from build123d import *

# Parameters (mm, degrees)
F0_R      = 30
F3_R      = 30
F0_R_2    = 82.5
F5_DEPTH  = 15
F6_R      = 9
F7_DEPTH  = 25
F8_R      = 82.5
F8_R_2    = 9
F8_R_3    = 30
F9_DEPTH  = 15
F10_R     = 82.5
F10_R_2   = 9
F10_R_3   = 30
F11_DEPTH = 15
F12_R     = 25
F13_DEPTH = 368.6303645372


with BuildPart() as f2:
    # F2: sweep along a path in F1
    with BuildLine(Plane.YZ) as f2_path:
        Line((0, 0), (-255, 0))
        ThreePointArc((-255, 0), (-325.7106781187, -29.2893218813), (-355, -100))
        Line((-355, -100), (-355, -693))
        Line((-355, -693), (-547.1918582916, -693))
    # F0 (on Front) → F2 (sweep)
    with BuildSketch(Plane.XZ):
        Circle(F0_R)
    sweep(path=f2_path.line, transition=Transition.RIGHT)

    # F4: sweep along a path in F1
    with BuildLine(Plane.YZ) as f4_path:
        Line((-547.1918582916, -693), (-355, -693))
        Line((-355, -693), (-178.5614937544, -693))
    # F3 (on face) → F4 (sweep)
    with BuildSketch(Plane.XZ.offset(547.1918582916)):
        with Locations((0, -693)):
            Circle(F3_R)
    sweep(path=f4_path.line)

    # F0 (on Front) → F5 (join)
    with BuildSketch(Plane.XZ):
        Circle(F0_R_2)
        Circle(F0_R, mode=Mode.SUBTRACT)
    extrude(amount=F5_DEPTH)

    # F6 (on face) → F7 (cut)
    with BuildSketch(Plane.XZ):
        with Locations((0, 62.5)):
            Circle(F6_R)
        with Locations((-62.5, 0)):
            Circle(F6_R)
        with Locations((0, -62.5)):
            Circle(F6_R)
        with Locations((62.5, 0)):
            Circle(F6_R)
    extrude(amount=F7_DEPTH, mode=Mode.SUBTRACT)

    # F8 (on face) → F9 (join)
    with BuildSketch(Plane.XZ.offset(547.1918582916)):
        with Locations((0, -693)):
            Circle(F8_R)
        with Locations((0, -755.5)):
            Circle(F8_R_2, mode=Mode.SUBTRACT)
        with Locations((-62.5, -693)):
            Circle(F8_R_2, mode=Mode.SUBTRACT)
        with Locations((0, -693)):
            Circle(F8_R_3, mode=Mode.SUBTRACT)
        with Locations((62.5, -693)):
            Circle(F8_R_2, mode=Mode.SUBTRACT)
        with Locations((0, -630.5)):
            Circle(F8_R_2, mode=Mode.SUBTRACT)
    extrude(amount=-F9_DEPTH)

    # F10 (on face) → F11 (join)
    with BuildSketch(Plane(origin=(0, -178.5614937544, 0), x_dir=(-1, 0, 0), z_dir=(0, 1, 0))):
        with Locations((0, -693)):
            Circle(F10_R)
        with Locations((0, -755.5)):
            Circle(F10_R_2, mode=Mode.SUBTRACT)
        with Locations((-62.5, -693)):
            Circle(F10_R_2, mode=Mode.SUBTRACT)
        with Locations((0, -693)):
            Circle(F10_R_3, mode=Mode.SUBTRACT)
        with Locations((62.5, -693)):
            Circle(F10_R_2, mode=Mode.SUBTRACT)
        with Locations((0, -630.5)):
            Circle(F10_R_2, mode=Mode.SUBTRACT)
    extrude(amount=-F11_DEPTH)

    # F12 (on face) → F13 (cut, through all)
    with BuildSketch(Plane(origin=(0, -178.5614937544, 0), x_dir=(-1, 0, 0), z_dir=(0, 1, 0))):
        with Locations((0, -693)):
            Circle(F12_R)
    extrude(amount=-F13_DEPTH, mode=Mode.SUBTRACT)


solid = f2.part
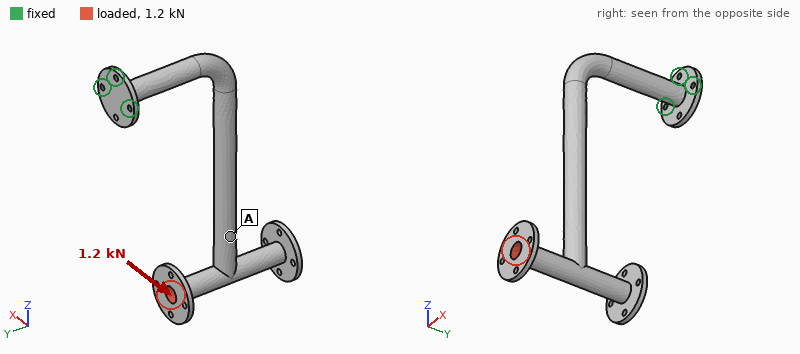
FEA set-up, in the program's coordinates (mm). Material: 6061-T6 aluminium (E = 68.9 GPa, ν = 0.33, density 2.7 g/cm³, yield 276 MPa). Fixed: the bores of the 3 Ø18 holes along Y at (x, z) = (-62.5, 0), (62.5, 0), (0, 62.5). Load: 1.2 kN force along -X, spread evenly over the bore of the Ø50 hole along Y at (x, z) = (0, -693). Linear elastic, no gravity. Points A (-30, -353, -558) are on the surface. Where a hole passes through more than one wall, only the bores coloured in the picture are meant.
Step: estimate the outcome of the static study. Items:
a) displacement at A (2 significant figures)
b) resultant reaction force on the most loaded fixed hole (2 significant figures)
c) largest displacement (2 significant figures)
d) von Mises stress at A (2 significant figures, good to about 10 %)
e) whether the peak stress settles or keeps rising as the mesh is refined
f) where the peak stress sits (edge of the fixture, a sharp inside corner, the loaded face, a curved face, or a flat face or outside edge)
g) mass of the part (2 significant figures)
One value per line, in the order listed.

7.1 mm
6.9 kN
11 mm
7.9 MPa
keeps rising
edge of the fixture
10 kg
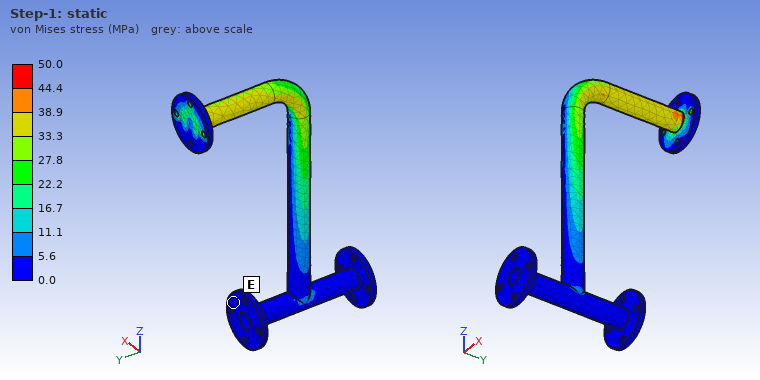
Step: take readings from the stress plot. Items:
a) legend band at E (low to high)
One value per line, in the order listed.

0.0 to 5.6 MPa
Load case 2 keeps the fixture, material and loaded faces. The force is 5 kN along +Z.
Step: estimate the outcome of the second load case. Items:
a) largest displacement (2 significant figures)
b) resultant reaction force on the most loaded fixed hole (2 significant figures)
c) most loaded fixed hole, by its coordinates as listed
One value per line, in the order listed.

11 mm
24 kN
(0, 62.5)
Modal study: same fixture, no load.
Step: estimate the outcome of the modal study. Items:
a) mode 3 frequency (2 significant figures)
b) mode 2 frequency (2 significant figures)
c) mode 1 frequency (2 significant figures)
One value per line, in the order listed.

110 Hz
30 Hz
29 Hz
